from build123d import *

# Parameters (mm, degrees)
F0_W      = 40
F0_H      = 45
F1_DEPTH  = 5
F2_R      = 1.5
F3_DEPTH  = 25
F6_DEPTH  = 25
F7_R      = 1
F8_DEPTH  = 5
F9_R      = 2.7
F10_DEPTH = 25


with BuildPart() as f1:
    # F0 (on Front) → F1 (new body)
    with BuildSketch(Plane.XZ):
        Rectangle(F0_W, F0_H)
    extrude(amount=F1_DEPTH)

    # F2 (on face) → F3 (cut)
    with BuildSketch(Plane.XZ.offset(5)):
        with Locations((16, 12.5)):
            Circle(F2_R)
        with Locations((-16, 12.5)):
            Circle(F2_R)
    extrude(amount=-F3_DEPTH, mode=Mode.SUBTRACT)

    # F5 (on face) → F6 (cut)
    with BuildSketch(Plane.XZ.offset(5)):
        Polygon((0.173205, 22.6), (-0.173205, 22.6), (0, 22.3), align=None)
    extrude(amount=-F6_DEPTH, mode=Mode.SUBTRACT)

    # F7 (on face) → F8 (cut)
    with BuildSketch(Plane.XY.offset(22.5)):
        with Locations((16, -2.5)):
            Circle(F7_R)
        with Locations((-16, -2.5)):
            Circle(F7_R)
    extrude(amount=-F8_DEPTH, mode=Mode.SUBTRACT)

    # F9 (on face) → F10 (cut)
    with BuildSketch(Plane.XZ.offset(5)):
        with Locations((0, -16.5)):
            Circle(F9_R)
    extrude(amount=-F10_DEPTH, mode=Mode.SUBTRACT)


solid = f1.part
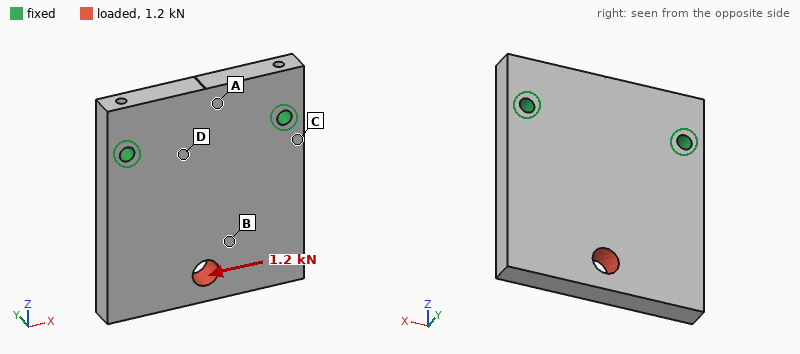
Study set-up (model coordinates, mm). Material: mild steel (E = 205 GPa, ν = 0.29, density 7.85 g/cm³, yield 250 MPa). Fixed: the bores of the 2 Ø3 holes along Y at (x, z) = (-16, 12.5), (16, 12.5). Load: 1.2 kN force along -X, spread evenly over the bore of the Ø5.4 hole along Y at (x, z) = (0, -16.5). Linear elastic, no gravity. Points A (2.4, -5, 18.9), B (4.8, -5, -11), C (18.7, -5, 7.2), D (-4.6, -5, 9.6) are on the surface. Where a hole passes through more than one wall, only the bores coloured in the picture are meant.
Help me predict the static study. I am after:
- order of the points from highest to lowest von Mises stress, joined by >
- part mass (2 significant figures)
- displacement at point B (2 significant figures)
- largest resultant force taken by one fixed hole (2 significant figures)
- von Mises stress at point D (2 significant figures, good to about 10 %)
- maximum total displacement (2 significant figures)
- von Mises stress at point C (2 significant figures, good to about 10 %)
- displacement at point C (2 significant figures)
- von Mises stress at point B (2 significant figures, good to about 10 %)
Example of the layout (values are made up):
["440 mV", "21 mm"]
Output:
["C > B > D > A", "69 g", "3.6 µm", "1.2 kN", "7.3 MPa", "5.8 µm", "20 MPa", "1.1 µm", "14 MPa"]
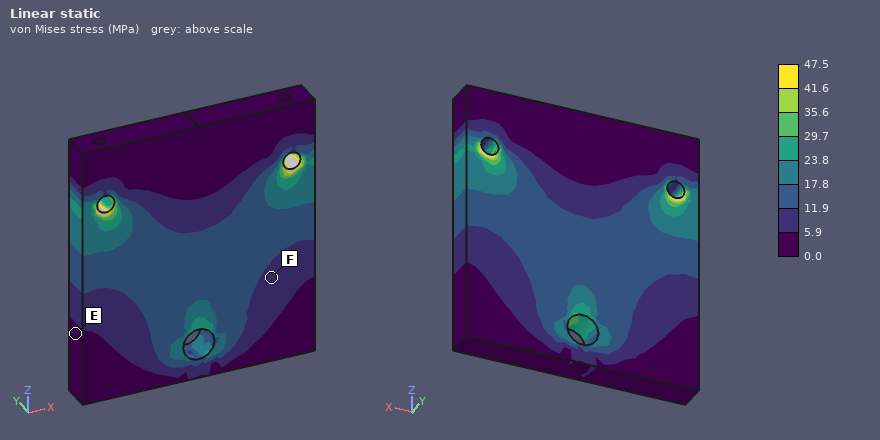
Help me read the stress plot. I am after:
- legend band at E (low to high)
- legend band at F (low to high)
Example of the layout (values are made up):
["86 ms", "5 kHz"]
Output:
["0.0 to 5.9 MPa", "5.9 to 11.9 MPa"]
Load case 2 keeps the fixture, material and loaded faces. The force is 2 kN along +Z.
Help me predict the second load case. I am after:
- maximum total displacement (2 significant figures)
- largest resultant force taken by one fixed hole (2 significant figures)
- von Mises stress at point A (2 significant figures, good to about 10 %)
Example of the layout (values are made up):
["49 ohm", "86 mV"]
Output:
["3.9 µm", "1.0 kN", "5.5 MPa"]
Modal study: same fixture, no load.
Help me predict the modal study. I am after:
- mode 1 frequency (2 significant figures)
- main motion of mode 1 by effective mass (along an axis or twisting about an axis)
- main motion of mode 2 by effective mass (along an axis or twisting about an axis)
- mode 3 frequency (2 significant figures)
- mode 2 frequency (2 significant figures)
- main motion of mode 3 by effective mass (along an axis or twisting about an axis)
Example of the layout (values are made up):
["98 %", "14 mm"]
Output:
["2900 Hz", "along Y", "twisting about Z", "16 kHz", "7100 Hz", "along X"]
